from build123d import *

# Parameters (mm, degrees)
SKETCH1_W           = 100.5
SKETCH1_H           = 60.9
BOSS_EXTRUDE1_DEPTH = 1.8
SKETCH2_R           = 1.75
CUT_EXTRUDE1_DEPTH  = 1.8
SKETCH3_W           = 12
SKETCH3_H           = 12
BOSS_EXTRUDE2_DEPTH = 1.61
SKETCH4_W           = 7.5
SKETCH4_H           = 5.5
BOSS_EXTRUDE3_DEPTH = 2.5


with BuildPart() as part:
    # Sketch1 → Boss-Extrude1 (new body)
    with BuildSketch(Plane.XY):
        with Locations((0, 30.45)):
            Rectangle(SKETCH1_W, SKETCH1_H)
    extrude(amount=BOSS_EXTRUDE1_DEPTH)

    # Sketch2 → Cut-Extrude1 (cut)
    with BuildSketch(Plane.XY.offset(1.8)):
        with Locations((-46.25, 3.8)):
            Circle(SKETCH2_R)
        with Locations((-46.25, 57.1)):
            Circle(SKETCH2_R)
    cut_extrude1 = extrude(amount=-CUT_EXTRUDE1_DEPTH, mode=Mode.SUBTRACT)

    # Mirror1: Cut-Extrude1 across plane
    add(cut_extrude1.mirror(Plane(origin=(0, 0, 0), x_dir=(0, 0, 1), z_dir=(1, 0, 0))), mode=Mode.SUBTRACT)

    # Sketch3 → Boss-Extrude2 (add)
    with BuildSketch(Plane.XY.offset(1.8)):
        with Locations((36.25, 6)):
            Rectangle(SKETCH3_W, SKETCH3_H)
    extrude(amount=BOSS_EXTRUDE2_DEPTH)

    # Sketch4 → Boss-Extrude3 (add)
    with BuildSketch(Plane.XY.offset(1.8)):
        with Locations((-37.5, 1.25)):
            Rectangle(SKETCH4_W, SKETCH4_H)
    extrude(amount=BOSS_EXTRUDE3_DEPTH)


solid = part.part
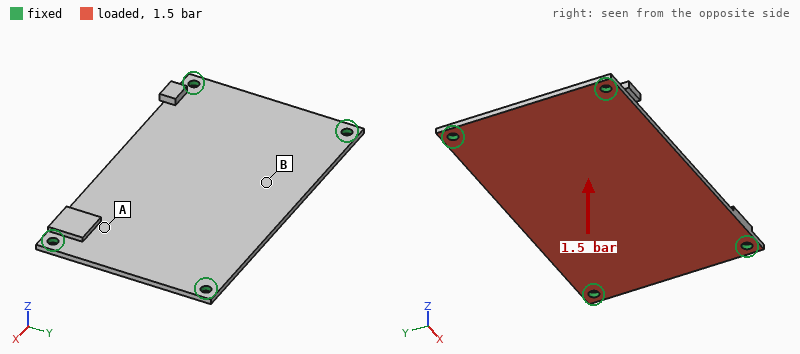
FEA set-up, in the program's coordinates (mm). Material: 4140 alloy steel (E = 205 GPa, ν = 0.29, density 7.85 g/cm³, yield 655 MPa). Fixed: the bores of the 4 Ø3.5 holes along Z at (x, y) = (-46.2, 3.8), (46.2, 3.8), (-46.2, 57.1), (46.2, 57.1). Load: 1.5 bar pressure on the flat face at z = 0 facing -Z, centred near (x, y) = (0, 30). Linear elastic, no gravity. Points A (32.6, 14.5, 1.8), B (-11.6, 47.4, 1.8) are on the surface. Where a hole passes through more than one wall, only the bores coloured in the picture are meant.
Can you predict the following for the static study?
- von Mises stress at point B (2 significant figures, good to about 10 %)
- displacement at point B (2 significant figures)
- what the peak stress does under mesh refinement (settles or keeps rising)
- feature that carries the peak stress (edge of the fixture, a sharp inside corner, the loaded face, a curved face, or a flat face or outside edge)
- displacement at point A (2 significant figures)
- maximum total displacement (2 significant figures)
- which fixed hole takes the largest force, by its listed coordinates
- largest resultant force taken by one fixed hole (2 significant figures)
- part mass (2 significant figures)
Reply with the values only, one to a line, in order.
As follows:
92 MPa
0.35 mm
keeps rising
edge of the fixture
0.14 mm
0.39 mm
(46.2, 3.8)
270 N
89 g
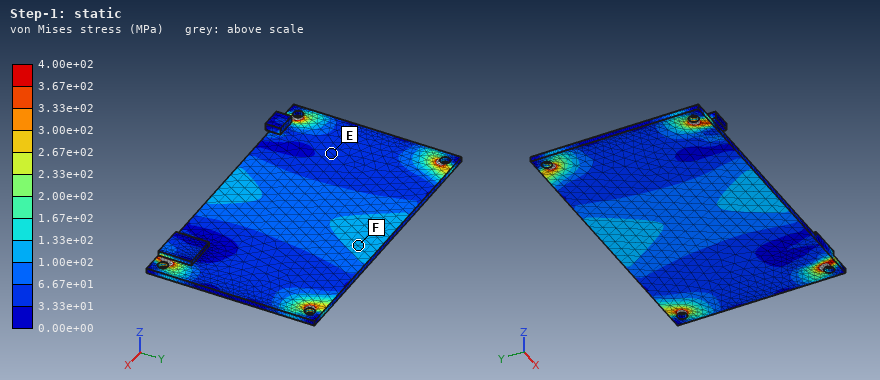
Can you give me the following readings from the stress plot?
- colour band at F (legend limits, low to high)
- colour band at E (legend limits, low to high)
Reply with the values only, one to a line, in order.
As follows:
1.00e+02 to 1.33e+02 MPa
3.33e+01 to 6.67e+01 MPa
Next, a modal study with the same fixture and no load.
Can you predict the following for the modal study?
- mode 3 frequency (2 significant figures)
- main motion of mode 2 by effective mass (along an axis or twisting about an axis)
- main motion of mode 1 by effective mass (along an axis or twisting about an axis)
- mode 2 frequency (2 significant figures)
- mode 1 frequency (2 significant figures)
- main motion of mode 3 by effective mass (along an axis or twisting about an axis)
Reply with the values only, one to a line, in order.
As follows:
2500 Hz
twisting about X
along Z
1600 Hz
960 Hz
twisting about Y
